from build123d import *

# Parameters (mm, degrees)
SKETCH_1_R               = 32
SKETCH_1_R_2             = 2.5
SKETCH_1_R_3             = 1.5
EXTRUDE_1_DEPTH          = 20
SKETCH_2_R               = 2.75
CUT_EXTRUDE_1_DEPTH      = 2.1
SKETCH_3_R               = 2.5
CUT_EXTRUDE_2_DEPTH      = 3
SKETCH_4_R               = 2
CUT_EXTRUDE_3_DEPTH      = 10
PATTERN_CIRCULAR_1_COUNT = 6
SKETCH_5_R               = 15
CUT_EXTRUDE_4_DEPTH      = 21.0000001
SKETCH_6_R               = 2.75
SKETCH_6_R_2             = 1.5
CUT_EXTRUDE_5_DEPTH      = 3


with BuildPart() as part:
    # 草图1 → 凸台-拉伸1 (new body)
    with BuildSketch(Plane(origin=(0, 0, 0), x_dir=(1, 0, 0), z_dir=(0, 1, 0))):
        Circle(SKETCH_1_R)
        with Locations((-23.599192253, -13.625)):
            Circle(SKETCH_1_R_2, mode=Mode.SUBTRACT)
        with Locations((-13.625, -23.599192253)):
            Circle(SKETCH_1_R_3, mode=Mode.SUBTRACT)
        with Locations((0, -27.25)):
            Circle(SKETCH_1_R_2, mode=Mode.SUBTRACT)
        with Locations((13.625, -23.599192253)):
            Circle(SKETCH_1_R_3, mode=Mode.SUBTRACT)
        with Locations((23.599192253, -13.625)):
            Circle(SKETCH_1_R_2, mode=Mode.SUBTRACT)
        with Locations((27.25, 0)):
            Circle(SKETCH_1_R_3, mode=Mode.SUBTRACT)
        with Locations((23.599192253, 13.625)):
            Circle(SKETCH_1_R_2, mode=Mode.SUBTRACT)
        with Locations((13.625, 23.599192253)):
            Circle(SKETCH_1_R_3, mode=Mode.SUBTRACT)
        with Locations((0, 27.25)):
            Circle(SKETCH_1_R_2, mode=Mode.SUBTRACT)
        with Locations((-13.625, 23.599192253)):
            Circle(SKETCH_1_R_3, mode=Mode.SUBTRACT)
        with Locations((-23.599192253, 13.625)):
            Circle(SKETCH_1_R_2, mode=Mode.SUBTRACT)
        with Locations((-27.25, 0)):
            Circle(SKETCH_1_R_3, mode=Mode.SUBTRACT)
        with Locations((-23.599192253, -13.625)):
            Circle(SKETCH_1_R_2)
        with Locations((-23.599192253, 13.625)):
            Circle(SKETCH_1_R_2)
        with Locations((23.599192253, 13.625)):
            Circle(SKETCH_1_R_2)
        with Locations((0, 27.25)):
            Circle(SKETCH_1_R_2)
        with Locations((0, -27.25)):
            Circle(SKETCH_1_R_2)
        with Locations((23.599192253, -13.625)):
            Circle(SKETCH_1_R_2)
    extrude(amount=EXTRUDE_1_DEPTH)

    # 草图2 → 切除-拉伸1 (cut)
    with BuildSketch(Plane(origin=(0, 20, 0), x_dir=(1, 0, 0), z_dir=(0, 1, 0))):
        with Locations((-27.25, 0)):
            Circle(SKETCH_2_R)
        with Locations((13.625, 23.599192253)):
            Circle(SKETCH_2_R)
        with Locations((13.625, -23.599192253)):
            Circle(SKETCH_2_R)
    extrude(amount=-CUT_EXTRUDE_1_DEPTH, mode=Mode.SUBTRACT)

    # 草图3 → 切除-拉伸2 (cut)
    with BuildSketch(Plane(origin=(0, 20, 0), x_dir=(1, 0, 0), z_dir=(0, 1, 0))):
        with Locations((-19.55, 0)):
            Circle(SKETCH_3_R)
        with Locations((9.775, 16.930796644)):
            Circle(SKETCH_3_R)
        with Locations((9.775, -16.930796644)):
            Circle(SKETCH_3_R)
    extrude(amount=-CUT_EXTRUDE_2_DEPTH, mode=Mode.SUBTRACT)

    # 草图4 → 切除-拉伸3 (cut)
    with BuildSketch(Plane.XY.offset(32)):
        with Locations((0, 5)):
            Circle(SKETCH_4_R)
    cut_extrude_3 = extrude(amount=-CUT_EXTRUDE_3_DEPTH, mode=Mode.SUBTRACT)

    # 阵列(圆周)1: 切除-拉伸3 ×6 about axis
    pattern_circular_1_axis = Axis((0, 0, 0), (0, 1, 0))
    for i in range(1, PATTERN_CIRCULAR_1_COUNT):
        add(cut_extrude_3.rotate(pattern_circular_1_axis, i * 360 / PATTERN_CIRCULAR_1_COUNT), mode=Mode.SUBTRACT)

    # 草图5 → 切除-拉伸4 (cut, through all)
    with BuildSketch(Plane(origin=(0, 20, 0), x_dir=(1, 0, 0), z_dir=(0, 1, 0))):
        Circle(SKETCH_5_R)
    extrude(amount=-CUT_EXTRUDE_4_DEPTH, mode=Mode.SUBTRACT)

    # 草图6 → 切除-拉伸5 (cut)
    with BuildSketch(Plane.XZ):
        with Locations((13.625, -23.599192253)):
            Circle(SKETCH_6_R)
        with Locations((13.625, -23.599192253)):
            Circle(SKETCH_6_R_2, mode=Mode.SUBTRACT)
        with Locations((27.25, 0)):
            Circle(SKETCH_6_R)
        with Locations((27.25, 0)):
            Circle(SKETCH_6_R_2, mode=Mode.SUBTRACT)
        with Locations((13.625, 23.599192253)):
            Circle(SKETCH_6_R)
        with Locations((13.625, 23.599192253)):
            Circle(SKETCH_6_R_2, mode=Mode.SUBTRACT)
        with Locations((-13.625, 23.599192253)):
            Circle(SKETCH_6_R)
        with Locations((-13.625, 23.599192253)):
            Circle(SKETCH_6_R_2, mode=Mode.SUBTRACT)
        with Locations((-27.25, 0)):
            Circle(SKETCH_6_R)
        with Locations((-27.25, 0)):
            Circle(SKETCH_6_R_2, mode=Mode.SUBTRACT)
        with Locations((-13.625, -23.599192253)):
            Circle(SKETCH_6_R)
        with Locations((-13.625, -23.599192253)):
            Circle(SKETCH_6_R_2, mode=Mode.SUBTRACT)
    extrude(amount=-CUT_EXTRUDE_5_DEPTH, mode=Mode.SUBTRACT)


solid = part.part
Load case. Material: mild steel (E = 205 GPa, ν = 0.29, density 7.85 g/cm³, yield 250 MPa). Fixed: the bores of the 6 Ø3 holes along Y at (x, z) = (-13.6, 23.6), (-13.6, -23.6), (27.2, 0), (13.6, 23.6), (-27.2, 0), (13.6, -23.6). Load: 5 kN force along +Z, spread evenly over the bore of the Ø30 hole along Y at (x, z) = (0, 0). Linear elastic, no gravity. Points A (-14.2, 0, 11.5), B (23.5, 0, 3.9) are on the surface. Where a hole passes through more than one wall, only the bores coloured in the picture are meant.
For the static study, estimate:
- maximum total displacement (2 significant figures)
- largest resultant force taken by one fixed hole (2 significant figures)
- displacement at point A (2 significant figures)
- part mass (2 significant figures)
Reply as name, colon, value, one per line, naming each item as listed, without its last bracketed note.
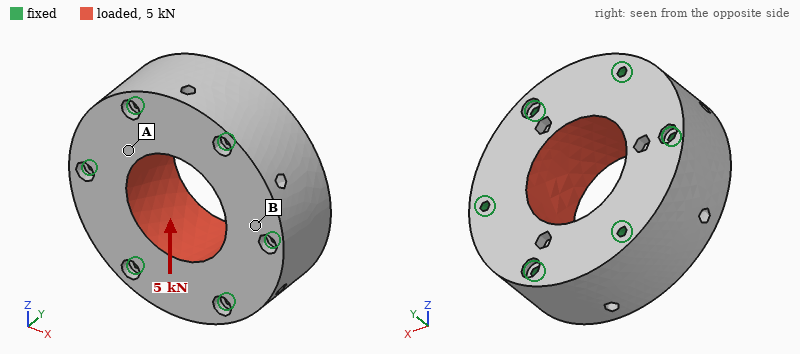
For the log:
maximum total displacement: 0.42 µm
largest resultant force taken by one fixed hole: 1000 N
displacement at point A: 0.26 µm
part mass: 380 g
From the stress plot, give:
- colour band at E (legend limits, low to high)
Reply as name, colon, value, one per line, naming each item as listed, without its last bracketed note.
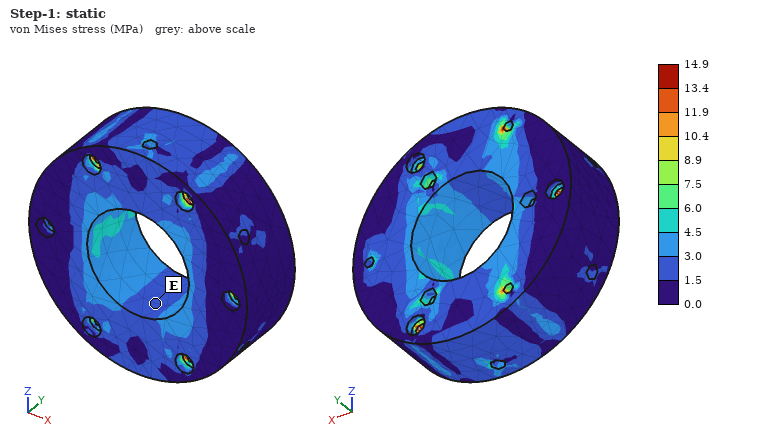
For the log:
colour band at E: 1.5 to 3.0 MPa
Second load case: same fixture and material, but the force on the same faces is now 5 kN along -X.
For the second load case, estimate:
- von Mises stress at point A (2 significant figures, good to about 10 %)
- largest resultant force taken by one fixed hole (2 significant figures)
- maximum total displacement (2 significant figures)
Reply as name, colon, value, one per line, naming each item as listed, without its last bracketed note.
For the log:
von Mises stress at point A: 1.8 MPa
largest resultant force taken by one fixed hole: 1.1 kN
maximum total displacement: 0.40 µm
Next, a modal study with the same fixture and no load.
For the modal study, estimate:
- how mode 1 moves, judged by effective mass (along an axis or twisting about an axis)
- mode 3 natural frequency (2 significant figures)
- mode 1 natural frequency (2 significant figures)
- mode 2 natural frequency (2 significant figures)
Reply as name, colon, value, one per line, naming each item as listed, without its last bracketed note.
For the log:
how mode 1 moves, judged by effective mass: along Y
mode 3 natural frequency: 41 kHz
mode 1 natural frequency: 34 kHz
mode 2 natural frequency: 40 kHz
